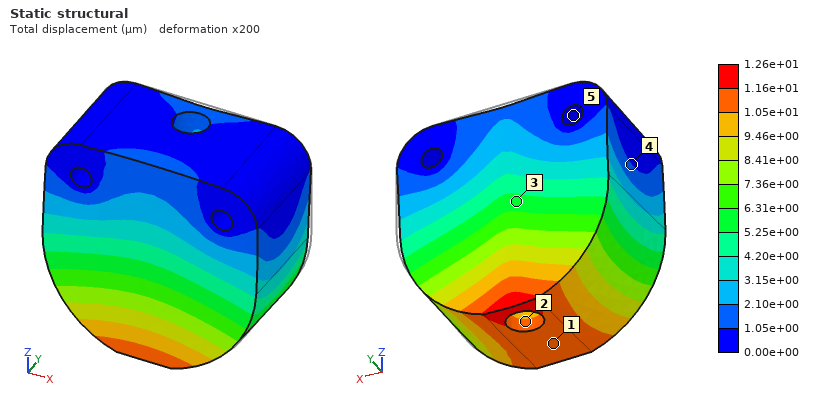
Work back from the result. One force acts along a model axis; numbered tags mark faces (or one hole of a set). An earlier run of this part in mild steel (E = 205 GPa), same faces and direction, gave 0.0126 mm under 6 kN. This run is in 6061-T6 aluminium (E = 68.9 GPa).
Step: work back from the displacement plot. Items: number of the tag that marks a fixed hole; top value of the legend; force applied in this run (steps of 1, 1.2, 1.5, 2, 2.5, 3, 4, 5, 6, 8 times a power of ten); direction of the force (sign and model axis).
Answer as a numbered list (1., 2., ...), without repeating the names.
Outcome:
1. 5
2. 1.26e+01 µm
3. 2 kN
4. -Y
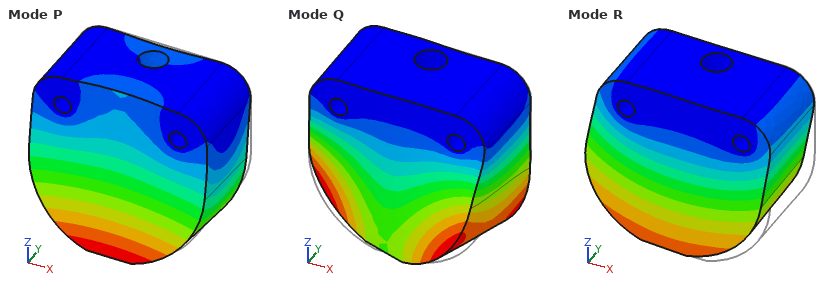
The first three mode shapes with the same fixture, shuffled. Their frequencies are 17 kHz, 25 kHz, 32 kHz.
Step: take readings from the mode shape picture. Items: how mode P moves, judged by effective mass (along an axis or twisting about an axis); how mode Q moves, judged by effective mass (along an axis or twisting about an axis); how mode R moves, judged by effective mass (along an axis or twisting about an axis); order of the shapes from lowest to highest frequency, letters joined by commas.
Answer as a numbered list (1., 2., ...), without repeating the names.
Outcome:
1. along Y
2. twisting about Z
3. along X
4. P, R, Q
